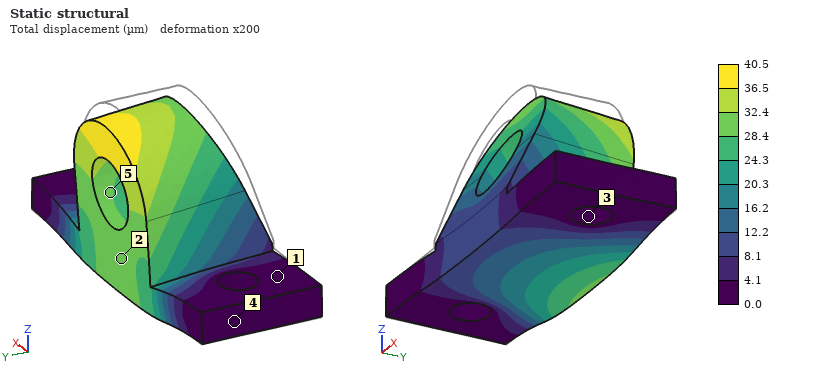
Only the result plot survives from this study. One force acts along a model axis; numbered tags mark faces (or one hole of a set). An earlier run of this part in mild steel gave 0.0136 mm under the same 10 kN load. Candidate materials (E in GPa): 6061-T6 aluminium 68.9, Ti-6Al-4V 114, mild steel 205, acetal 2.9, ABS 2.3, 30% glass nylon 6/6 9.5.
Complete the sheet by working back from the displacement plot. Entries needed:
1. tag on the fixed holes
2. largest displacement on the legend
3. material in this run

3
40.5 µm
6061-T6 aluminium
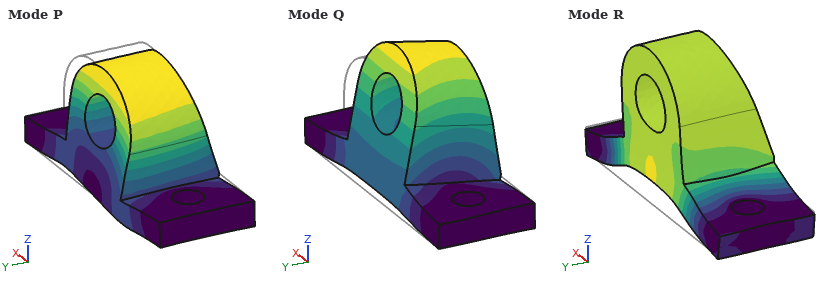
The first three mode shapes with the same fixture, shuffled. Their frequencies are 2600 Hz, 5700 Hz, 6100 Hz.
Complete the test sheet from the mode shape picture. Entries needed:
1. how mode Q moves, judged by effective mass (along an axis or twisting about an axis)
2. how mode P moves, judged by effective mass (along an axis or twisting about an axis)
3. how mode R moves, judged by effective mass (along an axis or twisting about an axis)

along Y
along X
along Z
